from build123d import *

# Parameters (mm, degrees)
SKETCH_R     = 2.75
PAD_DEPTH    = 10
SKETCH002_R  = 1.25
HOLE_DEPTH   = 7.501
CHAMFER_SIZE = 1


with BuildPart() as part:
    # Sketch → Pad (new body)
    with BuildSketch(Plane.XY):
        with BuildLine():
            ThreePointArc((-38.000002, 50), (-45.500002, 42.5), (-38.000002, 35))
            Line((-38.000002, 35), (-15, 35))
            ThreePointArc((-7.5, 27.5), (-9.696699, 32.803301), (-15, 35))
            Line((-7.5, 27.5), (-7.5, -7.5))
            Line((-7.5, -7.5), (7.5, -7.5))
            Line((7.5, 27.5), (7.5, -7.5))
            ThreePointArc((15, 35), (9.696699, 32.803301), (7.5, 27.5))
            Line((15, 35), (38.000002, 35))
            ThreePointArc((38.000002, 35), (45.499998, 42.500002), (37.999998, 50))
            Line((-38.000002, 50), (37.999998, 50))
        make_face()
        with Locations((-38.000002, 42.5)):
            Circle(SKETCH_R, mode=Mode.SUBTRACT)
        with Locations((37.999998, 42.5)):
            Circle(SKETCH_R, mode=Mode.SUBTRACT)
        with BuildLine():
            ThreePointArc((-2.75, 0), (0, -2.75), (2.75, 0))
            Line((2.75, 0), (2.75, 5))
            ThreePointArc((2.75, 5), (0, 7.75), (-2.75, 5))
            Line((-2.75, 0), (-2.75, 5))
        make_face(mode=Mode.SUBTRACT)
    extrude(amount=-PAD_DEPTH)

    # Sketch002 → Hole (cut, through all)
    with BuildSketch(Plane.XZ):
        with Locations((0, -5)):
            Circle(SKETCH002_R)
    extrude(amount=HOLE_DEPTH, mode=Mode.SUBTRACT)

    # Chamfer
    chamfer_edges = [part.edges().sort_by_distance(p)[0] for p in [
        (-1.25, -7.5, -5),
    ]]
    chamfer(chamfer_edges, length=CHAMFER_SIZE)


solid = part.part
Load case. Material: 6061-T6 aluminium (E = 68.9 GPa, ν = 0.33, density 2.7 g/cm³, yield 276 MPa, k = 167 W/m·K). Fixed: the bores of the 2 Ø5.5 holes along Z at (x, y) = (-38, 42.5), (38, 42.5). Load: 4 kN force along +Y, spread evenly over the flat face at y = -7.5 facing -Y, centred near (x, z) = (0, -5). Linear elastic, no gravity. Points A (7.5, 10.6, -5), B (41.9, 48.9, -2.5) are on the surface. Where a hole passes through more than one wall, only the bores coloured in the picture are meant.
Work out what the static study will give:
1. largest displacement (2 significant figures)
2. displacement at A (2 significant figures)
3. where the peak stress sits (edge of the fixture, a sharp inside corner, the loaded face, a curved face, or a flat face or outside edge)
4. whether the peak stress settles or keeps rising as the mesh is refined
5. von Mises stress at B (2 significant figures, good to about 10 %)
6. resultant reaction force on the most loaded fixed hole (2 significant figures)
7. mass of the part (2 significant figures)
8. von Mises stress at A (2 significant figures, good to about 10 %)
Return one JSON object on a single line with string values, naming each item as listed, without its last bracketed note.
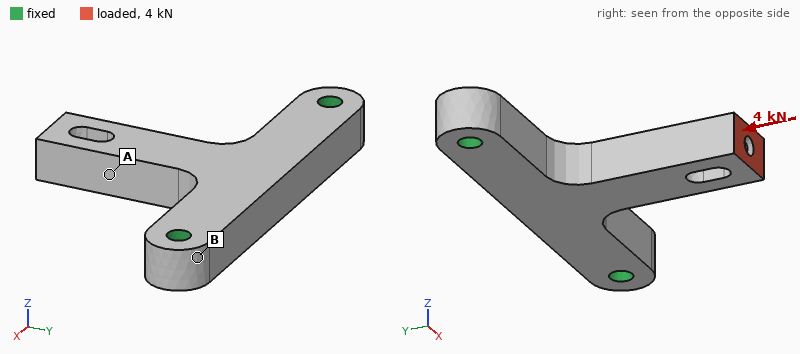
{"largest displacement": "79 µm", "displacement at A": "67 µm", "where the peak stress sits": "edge of the fixture", "whether the peak stress settles or keeps rising as the mesh is refined": "keeps rising", "von Mises stress at B": "16 MPa", "resultant reaction force on the most loaded fixed hole": "2.1 kN", "mass of the part": "51 g", "von Mises stress at A": "42 MPa"}
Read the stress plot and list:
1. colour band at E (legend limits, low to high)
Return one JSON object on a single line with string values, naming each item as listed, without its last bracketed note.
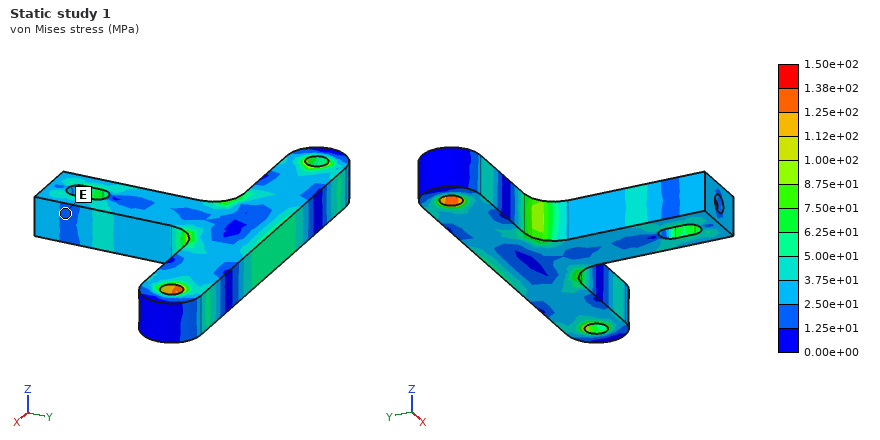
{"colour band at E": "1.25e+01 to 2.50e+01 MPa"}
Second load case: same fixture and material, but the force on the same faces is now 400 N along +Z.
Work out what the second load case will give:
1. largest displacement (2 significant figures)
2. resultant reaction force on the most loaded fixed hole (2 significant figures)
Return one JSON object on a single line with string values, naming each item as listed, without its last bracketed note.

{"largest displacement": "0.36 mm", "resultant reaction force on the most loaded fixed hole": "200 N"}
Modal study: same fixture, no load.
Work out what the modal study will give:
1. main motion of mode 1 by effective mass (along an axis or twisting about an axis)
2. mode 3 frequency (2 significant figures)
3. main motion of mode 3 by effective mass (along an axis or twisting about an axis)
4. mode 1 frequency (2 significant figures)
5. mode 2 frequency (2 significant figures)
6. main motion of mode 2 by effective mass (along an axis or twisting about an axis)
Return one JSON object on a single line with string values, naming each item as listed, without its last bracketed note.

{"main motion of mode 1 by effective mass": "along Z", "mode 3 frequency": "7400 Hz", "main motion of mode 3 by effective mass": "along Y", "mode 1 frequency": "2300 Hz", "mode 2 frequency": "5600 Hz", "main motion of mode 2 by effective mass": "along X"}
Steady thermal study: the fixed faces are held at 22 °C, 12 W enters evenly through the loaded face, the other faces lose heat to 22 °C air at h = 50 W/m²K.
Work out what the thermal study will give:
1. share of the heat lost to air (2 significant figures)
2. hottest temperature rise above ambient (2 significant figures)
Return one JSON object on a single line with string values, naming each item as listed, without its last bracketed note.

{"share of the heat lost to air": "21 %", "hottest temperature rise above ambient": "28 K"}
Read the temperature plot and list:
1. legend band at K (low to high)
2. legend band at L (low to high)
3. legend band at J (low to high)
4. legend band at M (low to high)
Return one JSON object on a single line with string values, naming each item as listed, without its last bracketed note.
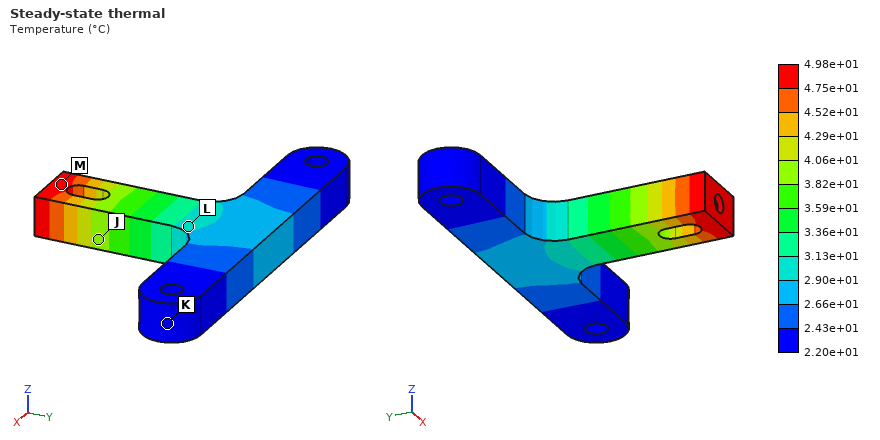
{"legend band at K": "2.20e+01 to 2.43e+01 °C", "legend band at L": "2.90e+01 to 3.13e+01 °C", "legend band at J": "3.82e+01 to 4.06e+01 °C", "legend band at M": "4.75e+01 to 4.98e+01 °C"}
